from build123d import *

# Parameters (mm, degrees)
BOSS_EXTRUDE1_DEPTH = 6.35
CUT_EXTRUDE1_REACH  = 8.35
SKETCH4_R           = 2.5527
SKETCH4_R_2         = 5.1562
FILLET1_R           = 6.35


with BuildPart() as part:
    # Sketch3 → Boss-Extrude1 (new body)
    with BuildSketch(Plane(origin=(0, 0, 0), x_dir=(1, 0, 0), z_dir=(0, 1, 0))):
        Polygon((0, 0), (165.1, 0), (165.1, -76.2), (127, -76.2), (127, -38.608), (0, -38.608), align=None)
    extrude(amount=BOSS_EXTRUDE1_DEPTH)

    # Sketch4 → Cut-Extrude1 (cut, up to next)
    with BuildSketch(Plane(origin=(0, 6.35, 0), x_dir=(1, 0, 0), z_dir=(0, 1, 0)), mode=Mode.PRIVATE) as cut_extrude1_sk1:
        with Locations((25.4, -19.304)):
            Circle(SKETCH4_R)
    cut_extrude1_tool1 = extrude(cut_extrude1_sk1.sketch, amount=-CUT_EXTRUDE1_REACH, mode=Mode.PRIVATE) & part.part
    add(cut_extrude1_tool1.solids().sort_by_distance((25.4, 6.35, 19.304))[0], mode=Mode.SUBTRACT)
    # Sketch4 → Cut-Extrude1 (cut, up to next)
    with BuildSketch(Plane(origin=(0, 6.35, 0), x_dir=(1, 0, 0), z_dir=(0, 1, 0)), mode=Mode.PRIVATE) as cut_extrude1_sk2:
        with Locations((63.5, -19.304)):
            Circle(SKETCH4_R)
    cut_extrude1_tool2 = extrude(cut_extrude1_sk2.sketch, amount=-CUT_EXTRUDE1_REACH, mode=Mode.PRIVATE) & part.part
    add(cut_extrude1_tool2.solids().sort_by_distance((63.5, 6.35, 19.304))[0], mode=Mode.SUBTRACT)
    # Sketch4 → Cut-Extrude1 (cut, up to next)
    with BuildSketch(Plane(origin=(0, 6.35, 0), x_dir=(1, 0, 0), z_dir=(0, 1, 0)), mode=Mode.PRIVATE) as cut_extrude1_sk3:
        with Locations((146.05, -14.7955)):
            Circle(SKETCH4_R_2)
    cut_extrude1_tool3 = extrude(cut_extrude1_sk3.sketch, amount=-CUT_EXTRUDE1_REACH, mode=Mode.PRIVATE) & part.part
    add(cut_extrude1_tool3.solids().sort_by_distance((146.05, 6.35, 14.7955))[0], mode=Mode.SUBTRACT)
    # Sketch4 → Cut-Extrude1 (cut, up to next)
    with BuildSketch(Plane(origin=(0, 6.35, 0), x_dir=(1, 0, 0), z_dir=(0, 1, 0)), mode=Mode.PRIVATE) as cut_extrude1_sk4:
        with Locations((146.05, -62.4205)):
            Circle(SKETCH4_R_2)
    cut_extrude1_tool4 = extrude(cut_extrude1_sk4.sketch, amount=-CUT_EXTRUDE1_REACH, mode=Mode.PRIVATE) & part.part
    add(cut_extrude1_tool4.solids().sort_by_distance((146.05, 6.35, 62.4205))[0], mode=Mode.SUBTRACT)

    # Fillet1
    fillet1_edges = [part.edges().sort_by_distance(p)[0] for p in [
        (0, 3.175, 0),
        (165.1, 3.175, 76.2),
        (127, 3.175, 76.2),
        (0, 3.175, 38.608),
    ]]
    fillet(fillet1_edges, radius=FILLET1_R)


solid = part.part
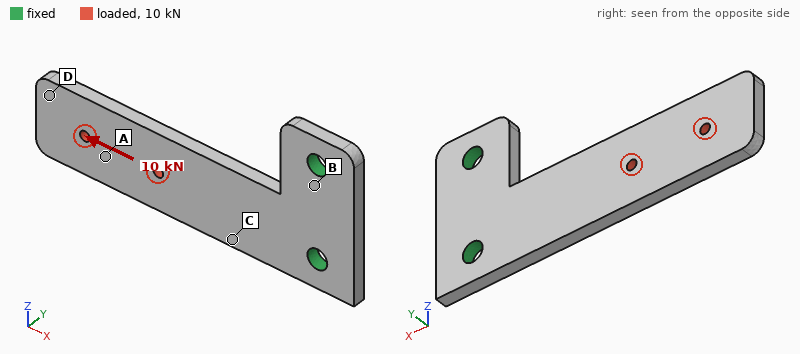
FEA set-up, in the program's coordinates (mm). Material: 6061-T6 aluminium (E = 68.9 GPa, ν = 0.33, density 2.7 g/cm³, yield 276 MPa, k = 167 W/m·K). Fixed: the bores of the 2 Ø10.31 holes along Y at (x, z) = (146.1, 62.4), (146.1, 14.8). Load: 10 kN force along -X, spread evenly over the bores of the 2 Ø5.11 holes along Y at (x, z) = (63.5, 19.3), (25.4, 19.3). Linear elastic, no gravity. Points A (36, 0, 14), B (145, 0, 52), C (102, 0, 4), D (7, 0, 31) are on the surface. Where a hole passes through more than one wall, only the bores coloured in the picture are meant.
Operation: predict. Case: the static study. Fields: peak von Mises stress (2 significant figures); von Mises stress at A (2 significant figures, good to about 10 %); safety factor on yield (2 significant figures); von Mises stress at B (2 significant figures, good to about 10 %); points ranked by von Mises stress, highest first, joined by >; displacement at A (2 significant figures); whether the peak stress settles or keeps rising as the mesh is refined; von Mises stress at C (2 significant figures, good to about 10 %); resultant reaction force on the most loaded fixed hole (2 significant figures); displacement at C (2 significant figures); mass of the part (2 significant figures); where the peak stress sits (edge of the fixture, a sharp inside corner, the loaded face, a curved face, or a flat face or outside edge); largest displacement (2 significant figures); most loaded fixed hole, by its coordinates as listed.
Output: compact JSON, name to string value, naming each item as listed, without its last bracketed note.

{"peak von Mises stress": "130 MPa", "von Mises stress at A": "27 MPa", "safety factor on yield": "2.2", "von Mises stress at B": "15 MPa", "points ranked by von Mises stress, highest first, joined by >": "C > A > B > D", "displacement at A": "61 µm", "whether the peak stress settles or keeps rising as the mesh is refined": "settles", "von Mises stress at C": "41 MPa", "resultant reaction force on the most loaded fixed hole": "8.8 kN", "displacement at C": "29 µm", "mass of the part": "130 g", "where the peak stress sits": "the loaded face", "largest displacement": "68 µm", "most loaded fixed hole, by its coordinates as listed": "(146.1, 14.8)"}
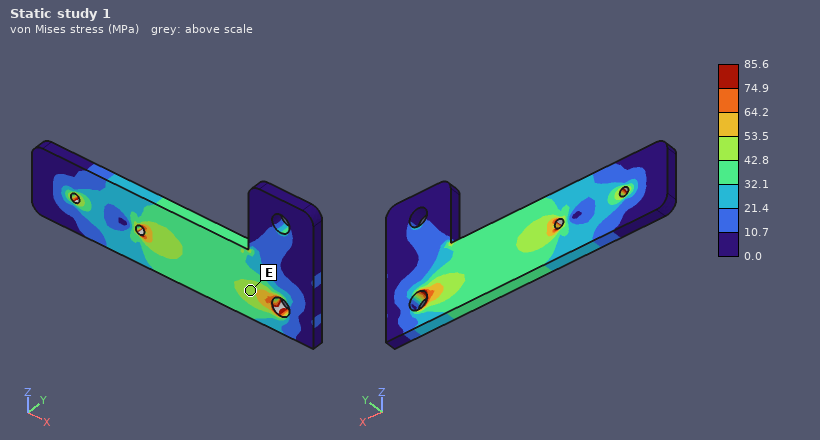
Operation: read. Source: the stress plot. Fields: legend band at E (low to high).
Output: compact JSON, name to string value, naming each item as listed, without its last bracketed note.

{"legend band at E": "42.8 to 53.5 MPa"}
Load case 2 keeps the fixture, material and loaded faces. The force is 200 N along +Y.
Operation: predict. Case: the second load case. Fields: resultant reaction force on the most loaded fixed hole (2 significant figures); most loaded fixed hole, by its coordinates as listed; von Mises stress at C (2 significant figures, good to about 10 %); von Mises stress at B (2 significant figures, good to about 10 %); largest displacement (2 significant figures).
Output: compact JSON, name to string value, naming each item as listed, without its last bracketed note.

{"resultant reaction force on the most loaded fixed hole": "230 N", "most loaded fixed hole, by its coordinates as listed": "(146.1, 14.8)", "von Mises stress at C": "44 MPa", "von Mises stress at B": "13 MPa", "largest displacement": "1.8 mm"}
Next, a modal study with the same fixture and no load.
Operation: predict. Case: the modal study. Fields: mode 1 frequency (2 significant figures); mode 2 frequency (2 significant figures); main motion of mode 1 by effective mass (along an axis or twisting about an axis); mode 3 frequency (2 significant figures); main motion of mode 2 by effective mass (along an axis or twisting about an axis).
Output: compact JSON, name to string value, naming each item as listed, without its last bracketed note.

{"mode 1 frequency": "260 Hz", "mode 2 frequency": "1400 Hz", "main motion of mode 1 by effective mass": "along Y", "mode 3 frequency": "1600 Hz", "main motion of mode 2 by effective mass": "along Z"}
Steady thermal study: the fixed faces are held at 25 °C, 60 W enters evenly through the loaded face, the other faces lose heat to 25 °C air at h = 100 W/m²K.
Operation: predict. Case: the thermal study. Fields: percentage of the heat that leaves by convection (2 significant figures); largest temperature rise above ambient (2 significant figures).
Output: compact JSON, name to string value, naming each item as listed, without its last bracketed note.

{"percentage of the heat that leaves by convection": "71 %", "largest temperature rise above ambient": "57 K"}
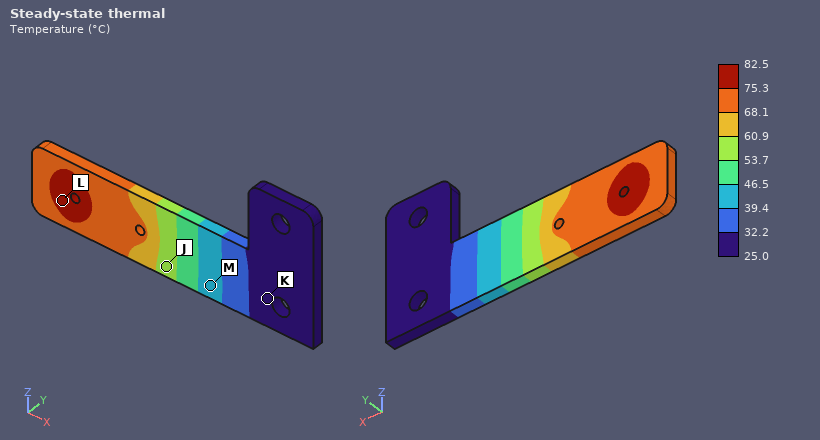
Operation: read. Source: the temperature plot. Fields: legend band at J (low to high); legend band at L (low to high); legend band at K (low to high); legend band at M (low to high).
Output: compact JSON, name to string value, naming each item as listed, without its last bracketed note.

{"legend band at J": "53.7 to 60.9 °C", "legend band at L": "75.3 to 82.5 °C", "legend band at K": "25.0 to 32.2 °C", "legend band at M": "39.4 to 46.5 °C"}
